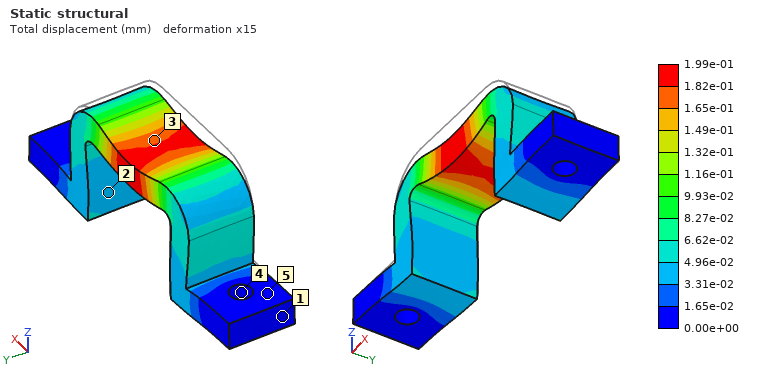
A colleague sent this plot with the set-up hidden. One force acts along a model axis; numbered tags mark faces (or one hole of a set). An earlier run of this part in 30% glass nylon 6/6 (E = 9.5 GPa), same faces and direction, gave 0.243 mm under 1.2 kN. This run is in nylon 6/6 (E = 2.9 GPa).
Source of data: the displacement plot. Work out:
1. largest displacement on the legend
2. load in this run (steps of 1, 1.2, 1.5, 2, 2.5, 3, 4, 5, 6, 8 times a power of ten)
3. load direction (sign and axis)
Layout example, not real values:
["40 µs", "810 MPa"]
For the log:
["1.99e-01 mm", "300 N", "-Z"]
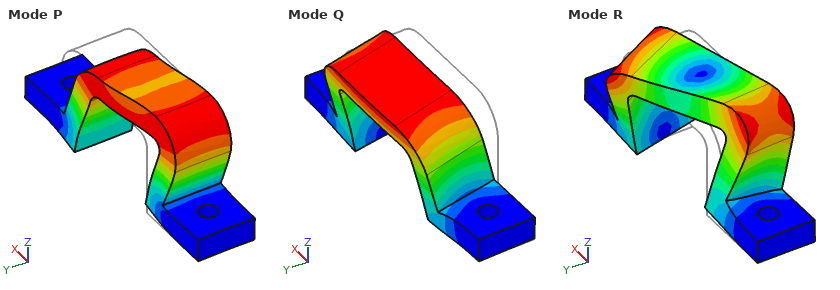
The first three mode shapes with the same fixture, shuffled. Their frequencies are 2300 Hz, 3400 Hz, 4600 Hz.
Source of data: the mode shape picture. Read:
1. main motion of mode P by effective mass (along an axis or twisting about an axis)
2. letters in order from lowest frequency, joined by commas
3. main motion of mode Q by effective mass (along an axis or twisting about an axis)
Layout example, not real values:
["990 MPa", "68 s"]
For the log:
["along X", "Q, P, R", "along Y"]
